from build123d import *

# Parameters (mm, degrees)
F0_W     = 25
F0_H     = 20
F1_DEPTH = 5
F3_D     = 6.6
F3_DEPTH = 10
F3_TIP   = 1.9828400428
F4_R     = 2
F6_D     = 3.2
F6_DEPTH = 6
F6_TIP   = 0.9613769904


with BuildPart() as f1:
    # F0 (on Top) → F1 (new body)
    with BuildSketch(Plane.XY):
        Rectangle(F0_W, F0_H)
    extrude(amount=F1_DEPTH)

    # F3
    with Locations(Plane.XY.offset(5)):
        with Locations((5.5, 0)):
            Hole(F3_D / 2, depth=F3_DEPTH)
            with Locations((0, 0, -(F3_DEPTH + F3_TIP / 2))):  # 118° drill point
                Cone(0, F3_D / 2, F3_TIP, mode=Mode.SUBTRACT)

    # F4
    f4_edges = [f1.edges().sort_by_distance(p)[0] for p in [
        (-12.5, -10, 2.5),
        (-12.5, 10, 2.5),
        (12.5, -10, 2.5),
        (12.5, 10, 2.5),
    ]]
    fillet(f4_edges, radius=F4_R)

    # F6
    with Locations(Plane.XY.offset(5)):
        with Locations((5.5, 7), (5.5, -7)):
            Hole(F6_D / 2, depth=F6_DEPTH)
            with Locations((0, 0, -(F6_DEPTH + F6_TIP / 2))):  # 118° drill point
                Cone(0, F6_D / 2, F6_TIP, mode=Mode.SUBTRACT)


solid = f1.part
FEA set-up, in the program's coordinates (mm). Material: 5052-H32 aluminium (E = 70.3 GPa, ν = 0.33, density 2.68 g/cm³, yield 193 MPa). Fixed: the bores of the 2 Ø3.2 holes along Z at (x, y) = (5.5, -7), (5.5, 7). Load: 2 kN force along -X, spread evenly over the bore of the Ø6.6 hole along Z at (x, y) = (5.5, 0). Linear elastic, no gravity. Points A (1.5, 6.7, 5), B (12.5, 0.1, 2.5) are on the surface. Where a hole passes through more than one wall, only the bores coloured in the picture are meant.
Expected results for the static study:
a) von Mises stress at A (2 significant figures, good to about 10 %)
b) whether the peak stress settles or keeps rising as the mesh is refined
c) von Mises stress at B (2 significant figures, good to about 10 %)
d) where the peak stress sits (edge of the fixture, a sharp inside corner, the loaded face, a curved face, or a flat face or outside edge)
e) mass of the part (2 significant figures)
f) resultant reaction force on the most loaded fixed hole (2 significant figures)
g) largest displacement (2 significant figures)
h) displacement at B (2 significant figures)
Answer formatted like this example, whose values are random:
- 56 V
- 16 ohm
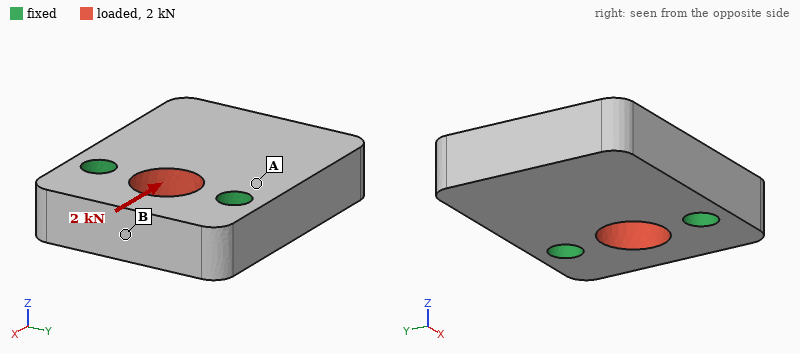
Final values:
- 13 MPa
- keeps rising
- 36 MPa
- edge of the fixture
- 6.0 g
- 1.0 kN
- 4.2 µm
- 3.3 µm
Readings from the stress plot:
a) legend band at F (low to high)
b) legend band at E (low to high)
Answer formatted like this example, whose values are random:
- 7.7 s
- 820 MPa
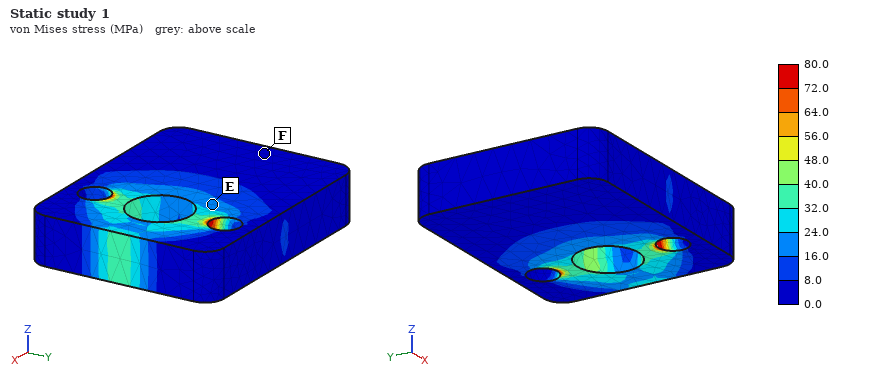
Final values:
- 0.0 to 8.0 MPa
- 16.0 to 24.0 MPa
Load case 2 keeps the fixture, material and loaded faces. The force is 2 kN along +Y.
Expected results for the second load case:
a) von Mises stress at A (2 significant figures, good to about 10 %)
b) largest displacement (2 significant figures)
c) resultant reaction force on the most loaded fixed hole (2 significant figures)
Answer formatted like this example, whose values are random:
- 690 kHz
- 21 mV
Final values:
- 8.3 MPa
- 2.8 µm
- 1.0 kN
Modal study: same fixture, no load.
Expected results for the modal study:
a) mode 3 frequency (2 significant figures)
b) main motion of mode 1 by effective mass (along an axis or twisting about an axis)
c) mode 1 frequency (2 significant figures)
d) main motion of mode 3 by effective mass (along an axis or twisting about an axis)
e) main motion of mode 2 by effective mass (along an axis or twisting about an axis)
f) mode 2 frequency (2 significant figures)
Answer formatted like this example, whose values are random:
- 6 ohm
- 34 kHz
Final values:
- 32 kHz
- along Z
- 12 kHz
- along Y
- twisting about X
- 25 kHz
